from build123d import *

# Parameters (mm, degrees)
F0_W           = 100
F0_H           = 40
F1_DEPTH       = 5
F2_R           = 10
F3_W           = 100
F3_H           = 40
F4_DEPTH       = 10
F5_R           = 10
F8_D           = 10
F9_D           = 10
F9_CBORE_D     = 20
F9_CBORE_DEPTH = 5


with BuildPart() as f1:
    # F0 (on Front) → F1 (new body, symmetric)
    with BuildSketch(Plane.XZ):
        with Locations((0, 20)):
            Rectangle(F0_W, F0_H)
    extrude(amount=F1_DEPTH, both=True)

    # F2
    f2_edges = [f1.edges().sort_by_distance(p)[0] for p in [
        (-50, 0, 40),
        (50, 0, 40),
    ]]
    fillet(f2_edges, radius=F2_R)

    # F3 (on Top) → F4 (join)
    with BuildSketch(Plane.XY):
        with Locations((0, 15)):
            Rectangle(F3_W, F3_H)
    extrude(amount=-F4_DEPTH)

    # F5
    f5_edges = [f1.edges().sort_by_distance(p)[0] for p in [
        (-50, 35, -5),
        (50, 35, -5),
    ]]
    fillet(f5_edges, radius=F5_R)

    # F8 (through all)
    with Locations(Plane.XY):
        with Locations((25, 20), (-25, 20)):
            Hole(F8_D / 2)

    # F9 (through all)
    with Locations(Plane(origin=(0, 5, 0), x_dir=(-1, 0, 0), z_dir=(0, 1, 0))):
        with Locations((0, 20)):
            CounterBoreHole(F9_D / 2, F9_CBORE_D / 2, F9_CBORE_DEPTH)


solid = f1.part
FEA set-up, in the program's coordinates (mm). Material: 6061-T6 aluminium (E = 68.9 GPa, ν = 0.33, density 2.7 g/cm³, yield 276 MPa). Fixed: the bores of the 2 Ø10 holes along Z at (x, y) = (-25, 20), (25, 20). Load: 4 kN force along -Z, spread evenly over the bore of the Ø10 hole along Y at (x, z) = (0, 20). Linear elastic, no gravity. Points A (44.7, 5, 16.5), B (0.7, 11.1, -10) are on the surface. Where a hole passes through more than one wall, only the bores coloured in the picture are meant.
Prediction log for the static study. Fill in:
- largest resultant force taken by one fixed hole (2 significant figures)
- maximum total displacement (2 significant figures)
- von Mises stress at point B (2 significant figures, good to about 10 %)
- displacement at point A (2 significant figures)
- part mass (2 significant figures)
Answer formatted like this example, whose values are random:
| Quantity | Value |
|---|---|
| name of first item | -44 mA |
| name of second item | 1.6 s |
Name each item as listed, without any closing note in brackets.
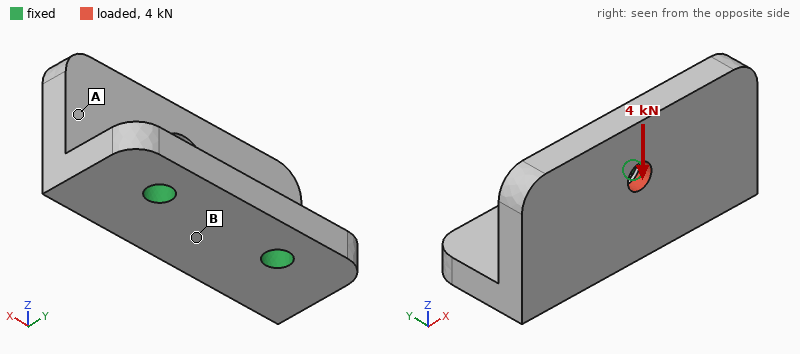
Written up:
| Quantity | Value |
|---|---|
| largest resultant force taken by one fixed hole | 2.0 kN |
| maximum total displacement | 0.11 mm |
| von Mises stress at point B | 19 MPa |
| displacement at point A | 0.041 mm |
| part mass | 200 g |
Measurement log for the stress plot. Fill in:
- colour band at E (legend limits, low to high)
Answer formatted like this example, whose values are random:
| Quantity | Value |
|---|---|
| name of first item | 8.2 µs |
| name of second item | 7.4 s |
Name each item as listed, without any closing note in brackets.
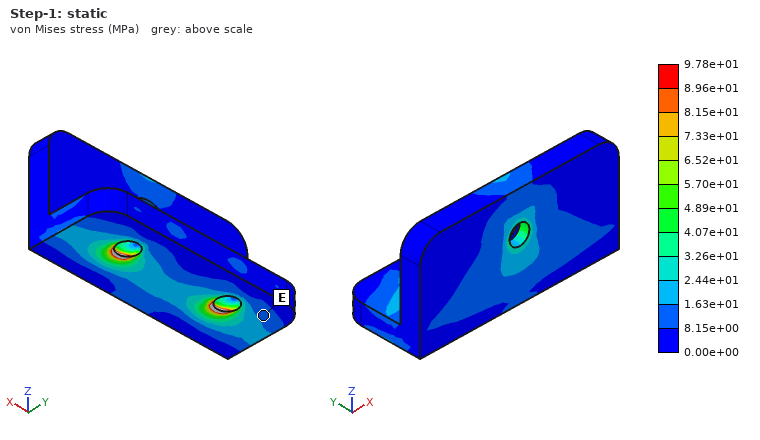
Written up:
| Quantity | Value |
|---|---|
| colour band at E | 8.15e+00 to 1.63e+01 MPa |
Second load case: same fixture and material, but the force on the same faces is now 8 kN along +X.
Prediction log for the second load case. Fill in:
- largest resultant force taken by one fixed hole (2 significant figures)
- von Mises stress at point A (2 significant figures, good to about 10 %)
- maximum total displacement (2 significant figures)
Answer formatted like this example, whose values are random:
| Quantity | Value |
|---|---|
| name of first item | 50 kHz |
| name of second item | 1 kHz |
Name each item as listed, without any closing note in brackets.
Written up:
| Quantity | Value |
|---|---|
| largest resultant force taken by one fixed hole | 5.9 kN |
| von Mises stress at point A | 13 MPa |
| maximum total displacement | 78 µm |
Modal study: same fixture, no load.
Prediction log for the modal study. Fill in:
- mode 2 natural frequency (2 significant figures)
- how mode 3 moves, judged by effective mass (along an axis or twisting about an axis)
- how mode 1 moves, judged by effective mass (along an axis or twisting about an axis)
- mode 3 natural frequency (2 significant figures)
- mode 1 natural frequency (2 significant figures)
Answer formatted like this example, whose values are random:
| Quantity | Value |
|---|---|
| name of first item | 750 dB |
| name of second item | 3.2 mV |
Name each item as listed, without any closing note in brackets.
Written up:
| Quantity | Value |
|---|---|
| mode 2 natural frequency | 3800 Hz |
| how mode 3 moves, judged by effective mass | along X |
| how mode 1 moves, judged by effective mass | along Y |
| mode 3 natural frequency | 6100 Hz |
| mode 1 natural frequency | 2500 Hz |
